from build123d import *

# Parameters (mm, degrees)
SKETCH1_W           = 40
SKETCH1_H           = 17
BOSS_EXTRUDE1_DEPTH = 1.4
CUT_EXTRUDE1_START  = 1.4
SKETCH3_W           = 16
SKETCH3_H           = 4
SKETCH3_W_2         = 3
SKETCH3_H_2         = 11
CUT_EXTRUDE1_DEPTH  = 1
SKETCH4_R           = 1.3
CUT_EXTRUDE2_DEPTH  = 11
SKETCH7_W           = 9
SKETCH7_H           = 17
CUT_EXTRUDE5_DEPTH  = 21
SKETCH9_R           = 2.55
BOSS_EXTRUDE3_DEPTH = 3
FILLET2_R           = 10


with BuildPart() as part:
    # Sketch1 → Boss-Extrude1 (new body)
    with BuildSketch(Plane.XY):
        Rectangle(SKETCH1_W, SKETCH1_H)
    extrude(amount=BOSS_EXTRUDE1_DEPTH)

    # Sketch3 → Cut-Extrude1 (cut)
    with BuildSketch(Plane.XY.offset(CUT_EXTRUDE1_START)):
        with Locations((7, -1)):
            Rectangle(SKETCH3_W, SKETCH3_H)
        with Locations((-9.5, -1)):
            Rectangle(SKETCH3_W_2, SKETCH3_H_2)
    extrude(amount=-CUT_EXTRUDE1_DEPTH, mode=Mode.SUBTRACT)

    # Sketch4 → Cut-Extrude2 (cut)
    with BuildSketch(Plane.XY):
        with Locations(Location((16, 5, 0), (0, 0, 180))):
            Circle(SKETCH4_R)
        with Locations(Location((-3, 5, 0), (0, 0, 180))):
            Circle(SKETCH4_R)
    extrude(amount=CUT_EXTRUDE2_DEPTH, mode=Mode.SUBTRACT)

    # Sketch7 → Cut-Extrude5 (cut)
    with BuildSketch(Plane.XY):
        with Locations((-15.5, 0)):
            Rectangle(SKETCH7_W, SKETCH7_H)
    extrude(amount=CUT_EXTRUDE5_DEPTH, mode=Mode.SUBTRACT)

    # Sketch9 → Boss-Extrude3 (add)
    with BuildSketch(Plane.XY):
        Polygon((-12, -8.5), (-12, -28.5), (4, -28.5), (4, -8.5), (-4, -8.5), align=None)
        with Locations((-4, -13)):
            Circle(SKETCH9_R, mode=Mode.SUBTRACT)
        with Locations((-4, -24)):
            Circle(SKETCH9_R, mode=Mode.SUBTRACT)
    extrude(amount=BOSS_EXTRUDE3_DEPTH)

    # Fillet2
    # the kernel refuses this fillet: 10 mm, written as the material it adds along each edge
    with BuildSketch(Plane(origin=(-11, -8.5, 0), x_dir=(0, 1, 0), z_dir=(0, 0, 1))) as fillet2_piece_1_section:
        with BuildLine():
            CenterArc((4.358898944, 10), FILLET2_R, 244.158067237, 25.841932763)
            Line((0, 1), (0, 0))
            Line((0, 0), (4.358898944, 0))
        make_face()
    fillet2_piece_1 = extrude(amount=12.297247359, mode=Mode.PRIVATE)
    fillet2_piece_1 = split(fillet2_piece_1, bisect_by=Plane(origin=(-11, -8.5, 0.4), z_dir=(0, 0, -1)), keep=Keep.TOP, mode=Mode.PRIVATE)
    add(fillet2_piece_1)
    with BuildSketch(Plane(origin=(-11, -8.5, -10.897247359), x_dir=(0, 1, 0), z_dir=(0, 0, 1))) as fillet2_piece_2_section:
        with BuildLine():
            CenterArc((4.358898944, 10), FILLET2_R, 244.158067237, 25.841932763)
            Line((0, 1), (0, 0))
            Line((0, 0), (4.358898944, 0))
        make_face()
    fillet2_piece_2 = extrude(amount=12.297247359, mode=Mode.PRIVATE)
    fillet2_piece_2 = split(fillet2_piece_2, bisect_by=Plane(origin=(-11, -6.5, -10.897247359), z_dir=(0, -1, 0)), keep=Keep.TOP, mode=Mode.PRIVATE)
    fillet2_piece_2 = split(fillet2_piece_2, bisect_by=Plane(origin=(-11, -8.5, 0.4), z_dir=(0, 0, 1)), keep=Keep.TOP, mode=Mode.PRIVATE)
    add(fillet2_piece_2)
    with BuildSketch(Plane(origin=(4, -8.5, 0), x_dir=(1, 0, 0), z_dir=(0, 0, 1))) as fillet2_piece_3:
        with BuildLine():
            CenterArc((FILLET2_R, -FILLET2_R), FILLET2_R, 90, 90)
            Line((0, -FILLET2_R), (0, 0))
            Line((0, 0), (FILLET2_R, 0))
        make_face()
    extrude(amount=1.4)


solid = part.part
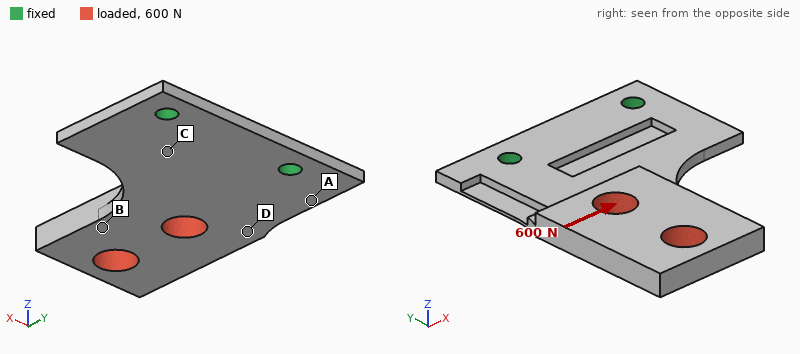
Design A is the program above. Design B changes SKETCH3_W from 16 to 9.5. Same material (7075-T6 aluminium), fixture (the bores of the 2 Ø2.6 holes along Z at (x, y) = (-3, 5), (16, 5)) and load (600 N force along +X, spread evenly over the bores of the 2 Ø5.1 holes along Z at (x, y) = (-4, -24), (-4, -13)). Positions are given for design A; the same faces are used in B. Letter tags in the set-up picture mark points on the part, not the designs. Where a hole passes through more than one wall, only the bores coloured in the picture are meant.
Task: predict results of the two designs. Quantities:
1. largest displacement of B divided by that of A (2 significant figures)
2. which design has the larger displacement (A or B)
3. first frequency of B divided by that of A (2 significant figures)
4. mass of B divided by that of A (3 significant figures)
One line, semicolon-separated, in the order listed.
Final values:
0.70; A; 1.1; 1.02
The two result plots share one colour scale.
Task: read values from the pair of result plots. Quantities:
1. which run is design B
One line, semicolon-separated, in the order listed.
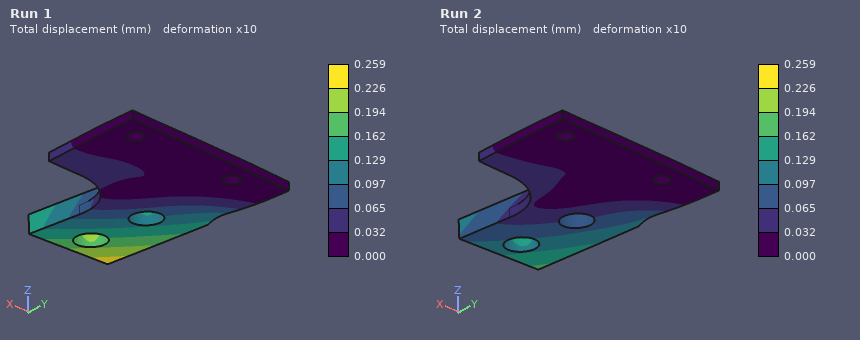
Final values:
Run 2
